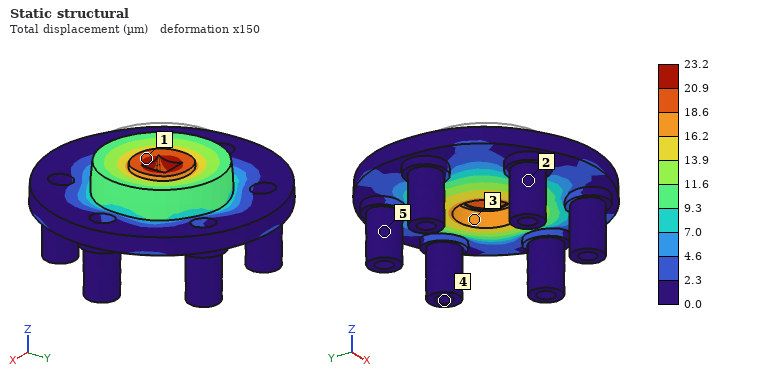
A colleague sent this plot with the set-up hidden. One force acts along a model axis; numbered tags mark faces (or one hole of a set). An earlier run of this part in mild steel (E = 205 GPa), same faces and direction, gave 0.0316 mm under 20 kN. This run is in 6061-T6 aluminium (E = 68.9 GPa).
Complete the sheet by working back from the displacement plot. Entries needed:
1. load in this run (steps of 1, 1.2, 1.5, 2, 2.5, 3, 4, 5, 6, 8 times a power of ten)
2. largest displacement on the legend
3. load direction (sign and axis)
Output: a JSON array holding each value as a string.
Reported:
["5 kN", "23.2 µm", "-Z"]
